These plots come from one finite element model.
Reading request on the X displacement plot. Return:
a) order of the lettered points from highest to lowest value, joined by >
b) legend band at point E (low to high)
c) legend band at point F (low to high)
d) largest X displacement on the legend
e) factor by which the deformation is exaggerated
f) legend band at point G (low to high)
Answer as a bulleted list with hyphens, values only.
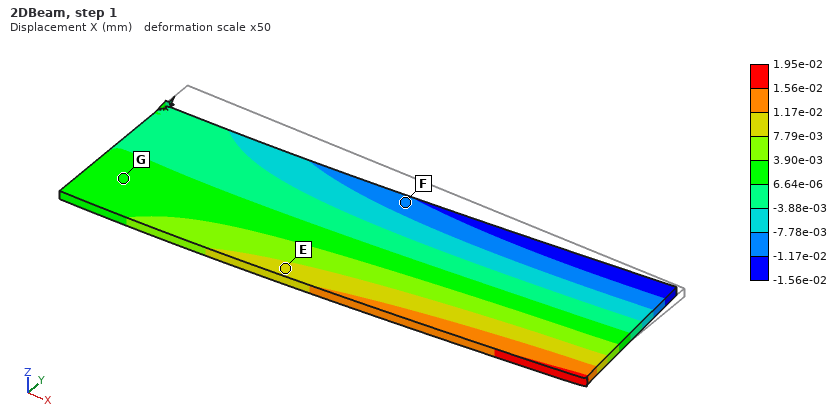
- E > G > F
- 7.79e-03 to 1.17e-02 mm
- -1.17e-02 to -7.78e-03 mm
- 1.95e-02 mm
- 50
- 6.64e-06 to 3.90e-03 mm
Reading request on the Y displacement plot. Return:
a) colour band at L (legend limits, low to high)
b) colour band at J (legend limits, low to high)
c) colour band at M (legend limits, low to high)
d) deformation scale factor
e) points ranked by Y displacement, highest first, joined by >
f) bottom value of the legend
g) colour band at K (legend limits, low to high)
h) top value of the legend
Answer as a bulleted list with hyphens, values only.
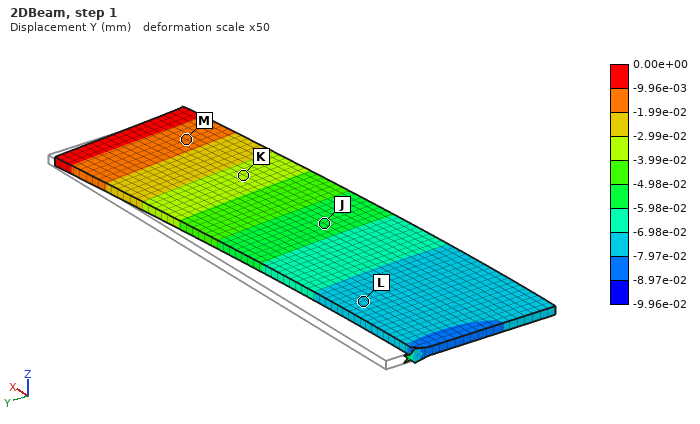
- -7.97e-02 to -6.98e-02 mm
- -5.98e-02 to -4.98e-02 mm
- -1.99e-02 to -9.96e-03 mm
- 50
- M > K > J > L
- -9.96e-02 mm
- -3.99e-02 to -2.99e-02 mm
- 0.00e+00 mm
